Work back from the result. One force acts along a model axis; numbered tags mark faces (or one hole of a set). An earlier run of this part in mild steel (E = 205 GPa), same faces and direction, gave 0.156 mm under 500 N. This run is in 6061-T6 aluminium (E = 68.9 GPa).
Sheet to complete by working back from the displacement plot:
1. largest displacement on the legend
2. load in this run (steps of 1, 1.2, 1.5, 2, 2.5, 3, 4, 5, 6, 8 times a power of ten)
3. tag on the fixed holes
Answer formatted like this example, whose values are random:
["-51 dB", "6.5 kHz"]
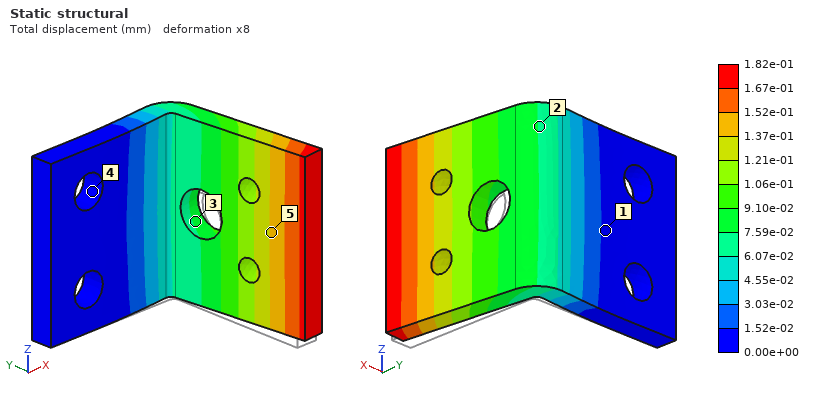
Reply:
["1.82e-01 mm", "200 N", "4"]
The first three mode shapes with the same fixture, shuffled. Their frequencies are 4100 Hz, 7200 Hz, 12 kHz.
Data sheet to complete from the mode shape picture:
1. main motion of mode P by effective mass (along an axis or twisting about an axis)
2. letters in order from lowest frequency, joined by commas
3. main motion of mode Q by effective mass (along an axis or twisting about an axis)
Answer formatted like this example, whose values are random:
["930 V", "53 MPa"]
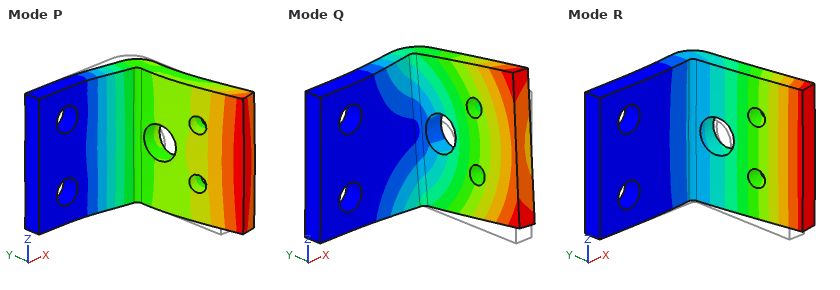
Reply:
["along Y", "R, Q, P", "along Z"]
